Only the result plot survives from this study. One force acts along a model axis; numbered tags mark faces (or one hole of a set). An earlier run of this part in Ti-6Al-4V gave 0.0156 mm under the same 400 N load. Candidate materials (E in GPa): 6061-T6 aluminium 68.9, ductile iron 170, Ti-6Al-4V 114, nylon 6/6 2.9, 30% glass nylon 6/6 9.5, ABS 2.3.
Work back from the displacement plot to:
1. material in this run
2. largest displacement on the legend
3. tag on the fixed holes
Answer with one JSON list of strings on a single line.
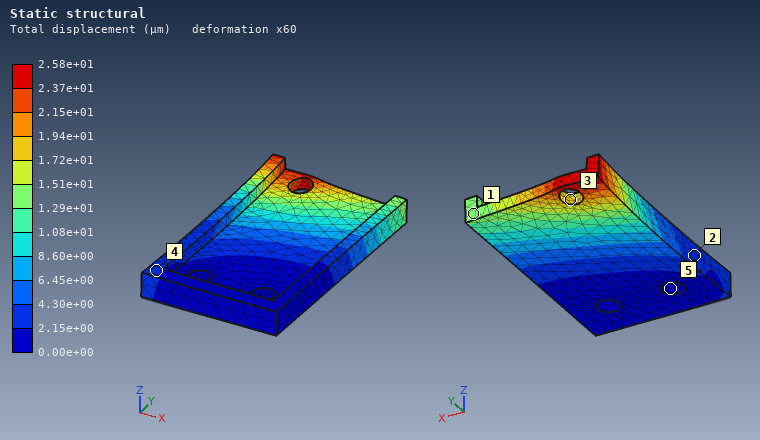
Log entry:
["6061-T6 aluminium", "2.58e+01 µm", "5"]
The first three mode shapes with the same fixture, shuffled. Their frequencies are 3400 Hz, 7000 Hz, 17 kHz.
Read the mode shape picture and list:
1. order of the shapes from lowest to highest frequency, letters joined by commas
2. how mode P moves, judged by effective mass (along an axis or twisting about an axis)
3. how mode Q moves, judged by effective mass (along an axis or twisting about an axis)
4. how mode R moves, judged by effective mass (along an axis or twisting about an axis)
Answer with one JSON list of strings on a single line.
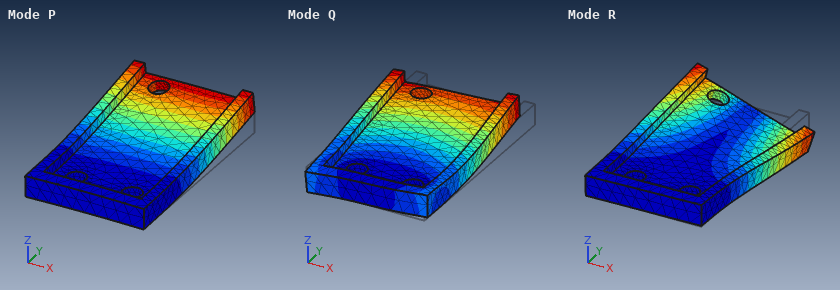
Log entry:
["P, R, Q", "along Z", "along X", "twisting about Y"]
